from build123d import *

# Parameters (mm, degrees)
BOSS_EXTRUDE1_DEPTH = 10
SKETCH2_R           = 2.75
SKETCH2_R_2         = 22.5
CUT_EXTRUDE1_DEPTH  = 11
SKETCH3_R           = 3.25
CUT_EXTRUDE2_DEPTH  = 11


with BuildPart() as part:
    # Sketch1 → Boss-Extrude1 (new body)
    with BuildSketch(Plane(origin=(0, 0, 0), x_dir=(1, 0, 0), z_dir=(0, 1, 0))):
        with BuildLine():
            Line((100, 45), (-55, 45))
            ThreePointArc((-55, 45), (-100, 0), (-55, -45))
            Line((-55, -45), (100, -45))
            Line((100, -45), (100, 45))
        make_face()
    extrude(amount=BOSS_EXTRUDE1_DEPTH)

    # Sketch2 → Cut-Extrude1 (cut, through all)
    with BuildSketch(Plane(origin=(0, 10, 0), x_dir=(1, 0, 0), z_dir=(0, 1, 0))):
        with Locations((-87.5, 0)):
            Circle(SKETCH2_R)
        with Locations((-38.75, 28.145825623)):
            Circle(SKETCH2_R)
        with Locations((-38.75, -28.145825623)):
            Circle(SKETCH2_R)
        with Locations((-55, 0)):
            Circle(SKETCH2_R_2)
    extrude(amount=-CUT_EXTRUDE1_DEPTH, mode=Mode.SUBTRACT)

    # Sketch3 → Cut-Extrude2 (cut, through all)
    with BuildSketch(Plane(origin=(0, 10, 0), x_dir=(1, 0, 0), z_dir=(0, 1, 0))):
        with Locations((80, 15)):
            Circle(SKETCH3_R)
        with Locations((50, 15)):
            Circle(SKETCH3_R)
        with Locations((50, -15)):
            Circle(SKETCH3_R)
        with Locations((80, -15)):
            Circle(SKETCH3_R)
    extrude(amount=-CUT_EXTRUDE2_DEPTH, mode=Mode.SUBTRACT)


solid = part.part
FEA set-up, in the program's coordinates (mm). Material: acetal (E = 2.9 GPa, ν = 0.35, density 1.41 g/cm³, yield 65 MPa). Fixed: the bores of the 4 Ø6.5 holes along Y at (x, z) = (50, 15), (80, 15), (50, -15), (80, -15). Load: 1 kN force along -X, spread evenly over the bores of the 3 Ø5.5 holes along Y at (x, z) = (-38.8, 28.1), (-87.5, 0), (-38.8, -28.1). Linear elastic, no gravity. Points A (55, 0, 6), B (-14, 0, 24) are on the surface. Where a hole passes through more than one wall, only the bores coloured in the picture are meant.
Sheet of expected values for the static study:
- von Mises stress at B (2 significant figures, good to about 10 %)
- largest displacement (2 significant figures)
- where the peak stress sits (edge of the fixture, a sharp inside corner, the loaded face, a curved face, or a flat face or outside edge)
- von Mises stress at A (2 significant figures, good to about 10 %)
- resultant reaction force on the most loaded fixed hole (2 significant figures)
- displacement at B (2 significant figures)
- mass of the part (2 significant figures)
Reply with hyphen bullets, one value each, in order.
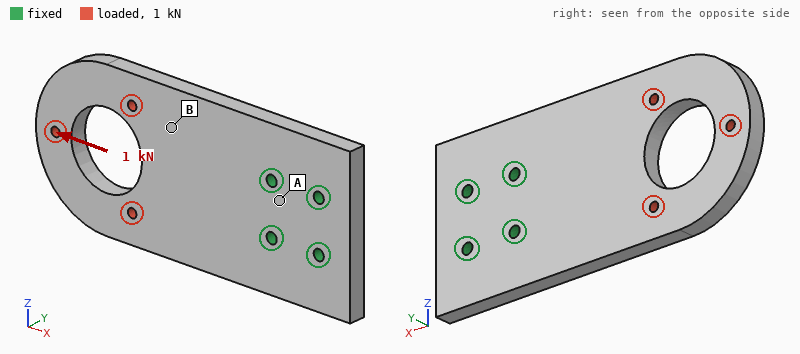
- 1.5 MPa
- 0.11 mm
- the loaded face
- 0.57 MPa
- 390 N
- 0.030 mm
- 220 g
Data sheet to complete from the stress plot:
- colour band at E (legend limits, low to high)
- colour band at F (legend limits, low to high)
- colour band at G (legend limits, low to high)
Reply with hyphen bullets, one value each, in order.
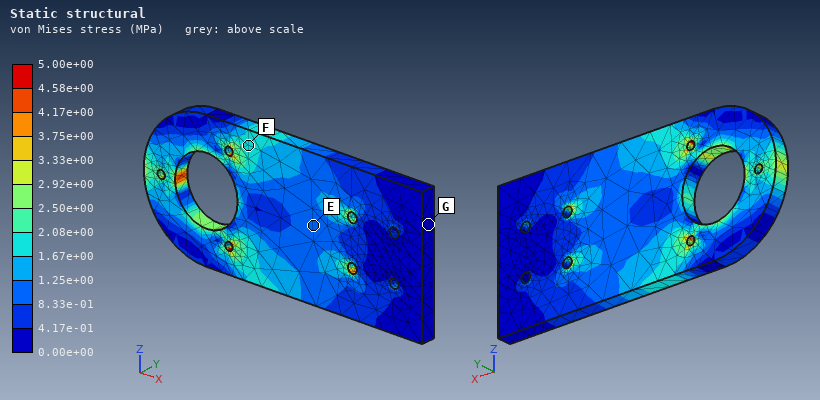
- 8.33e-01 to 1.25e+00 MPa
- 1.67e+00 to 2.08e+00 MPa
- 0.00e+00 to 4.17e-01 MPa
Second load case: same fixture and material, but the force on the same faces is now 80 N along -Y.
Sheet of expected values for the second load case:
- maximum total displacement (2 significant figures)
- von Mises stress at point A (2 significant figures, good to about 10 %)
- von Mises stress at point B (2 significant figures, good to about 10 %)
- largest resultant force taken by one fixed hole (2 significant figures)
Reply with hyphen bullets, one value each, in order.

- 2.5 mm
- 1.7 MPa
- 2.2 MPa
- 96 N
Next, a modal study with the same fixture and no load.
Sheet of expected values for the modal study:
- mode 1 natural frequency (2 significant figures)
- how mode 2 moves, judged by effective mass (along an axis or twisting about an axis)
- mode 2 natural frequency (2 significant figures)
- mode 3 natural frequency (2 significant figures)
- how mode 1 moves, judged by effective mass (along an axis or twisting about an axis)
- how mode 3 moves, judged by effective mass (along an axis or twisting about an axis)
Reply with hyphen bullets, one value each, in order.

- 130 Hz
- twisting about X
- 380 Hz
- 600 Hz
- along Y
- along Y
